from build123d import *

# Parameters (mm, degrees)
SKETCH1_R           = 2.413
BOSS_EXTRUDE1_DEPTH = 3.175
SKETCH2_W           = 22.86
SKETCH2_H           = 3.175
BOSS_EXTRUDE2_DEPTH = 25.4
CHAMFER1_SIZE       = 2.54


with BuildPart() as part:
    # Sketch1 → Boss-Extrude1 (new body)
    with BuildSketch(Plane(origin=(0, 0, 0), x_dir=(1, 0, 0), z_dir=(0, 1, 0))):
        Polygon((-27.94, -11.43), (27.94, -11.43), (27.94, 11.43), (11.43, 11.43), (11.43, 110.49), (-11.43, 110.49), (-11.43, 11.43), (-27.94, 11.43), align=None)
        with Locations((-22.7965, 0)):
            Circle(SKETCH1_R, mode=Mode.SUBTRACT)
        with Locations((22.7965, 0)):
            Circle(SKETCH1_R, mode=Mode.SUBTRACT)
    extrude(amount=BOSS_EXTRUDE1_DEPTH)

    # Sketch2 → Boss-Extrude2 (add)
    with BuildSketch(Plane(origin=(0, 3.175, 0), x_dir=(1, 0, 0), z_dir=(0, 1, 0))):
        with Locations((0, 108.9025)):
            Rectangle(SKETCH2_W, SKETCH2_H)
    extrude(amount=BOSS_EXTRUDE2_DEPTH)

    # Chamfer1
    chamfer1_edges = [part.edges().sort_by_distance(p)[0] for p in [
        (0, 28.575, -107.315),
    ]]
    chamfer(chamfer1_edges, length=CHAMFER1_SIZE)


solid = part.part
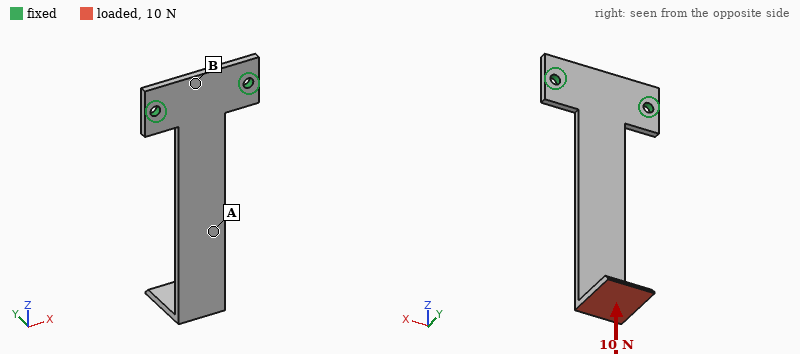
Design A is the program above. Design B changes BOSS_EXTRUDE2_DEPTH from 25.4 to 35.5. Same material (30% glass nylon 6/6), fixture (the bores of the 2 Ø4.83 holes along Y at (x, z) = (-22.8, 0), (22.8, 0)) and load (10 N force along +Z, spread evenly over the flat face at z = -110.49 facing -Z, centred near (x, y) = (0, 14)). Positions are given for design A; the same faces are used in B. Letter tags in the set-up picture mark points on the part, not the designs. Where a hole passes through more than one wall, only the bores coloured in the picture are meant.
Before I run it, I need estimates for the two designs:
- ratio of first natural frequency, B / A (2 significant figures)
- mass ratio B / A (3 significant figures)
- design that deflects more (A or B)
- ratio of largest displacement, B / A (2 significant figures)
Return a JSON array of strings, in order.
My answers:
["0.90", "1.06", "B", "1.5"]
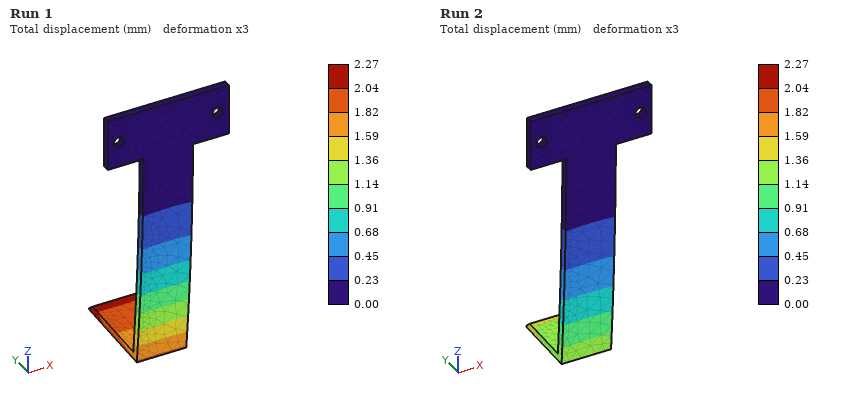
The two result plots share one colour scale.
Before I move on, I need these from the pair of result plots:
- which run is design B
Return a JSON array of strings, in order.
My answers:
["Run 1"]
